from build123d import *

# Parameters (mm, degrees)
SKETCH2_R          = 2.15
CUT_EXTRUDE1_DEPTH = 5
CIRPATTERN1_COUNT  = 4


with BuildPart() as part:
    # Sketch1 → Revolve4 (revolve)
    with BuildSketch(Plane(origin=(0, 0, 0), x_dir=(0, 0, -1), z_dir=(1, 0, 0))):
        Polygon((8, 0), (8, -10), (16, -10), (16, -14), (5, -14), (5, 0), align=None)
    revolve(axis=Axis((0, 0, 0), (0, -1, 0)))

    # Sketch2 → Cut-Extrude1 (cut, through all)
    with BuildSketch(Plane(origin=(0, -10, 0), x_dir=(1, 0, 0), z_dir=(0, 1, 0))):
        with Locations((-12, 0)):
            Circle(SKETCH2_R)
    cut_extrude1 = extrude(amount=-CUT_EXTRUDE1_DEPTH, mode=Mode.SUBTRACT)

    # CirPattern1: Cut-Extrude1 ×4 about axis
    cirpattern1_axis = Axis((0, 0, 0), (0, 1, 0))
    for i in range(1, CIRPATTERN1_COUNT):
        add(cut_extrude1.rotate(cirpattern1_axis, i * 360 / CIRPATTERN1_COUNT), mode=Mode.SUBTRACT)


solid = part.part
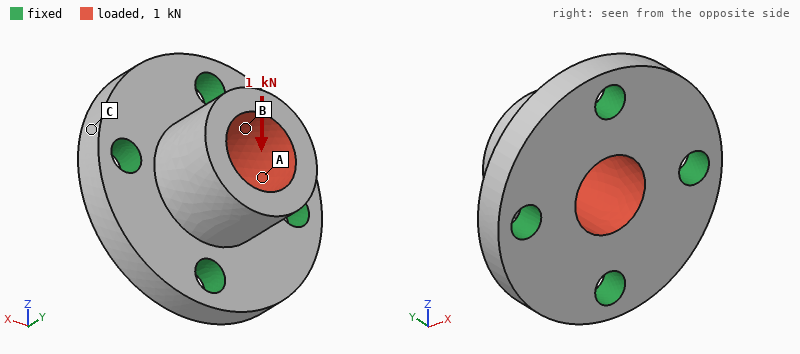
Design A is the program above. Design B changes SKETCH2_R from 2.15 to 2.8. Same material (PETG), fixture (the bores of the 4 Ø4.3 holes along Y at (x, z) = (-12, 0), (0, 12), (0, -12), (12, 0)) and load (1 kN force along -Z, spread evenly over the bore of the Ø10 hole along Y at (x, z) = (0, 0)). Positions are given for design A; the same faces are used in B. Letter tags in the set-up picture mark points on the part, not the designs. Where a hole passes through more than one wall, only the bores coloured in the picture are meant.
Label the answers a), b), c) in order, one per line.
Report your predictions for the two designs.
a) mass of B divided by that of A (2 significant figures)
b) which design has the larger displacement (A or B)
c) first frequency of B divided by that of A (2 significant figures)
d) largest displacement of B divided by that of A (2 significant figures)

a) 0.96
b) A
c) 1.1
d) 0.90
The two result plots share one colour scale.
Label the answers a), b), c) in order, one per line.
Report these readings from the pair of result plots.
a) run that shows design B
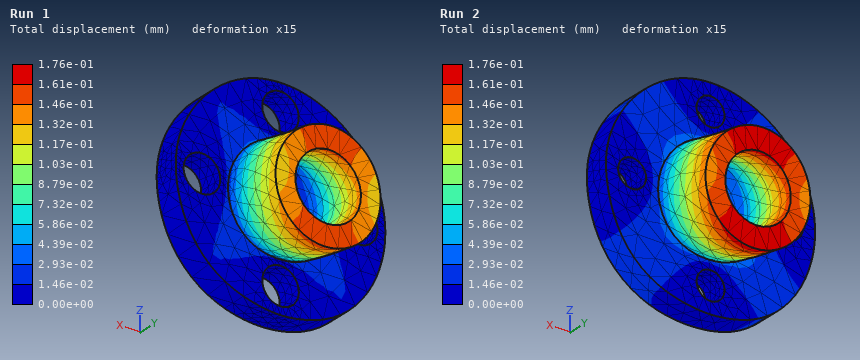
a) Run 1
